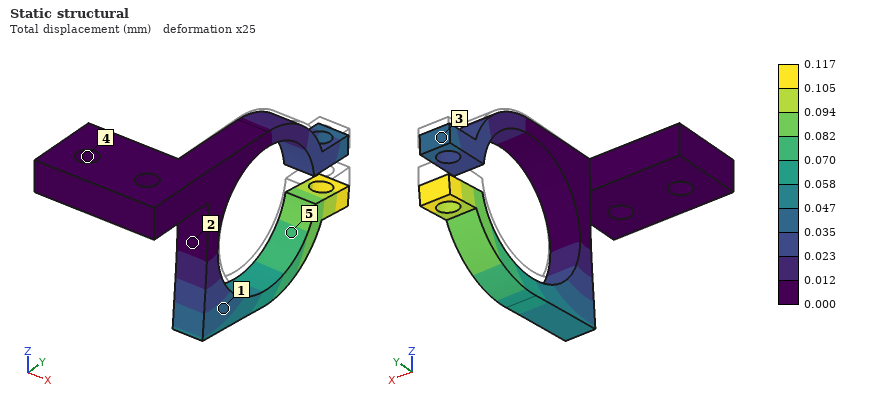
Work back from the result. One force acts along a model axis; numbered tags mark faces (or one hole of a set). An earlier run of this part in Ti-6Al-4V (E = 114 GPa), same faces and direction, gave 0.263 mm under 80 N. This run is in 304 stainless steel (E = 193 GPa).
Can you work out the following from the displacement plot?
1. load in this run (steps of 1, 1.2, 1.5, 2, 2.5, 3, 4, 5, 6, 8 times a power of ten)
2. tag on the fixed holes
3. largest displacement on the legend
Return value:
60 N
4
0.117 mm
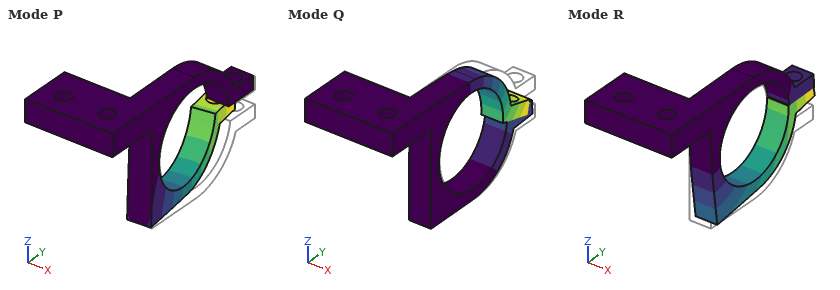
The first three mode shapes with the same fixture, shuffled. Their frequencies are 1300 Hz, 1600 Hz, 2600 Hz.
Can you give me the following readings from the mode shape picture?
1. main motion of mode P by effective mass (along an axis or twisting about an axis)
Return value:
along X
